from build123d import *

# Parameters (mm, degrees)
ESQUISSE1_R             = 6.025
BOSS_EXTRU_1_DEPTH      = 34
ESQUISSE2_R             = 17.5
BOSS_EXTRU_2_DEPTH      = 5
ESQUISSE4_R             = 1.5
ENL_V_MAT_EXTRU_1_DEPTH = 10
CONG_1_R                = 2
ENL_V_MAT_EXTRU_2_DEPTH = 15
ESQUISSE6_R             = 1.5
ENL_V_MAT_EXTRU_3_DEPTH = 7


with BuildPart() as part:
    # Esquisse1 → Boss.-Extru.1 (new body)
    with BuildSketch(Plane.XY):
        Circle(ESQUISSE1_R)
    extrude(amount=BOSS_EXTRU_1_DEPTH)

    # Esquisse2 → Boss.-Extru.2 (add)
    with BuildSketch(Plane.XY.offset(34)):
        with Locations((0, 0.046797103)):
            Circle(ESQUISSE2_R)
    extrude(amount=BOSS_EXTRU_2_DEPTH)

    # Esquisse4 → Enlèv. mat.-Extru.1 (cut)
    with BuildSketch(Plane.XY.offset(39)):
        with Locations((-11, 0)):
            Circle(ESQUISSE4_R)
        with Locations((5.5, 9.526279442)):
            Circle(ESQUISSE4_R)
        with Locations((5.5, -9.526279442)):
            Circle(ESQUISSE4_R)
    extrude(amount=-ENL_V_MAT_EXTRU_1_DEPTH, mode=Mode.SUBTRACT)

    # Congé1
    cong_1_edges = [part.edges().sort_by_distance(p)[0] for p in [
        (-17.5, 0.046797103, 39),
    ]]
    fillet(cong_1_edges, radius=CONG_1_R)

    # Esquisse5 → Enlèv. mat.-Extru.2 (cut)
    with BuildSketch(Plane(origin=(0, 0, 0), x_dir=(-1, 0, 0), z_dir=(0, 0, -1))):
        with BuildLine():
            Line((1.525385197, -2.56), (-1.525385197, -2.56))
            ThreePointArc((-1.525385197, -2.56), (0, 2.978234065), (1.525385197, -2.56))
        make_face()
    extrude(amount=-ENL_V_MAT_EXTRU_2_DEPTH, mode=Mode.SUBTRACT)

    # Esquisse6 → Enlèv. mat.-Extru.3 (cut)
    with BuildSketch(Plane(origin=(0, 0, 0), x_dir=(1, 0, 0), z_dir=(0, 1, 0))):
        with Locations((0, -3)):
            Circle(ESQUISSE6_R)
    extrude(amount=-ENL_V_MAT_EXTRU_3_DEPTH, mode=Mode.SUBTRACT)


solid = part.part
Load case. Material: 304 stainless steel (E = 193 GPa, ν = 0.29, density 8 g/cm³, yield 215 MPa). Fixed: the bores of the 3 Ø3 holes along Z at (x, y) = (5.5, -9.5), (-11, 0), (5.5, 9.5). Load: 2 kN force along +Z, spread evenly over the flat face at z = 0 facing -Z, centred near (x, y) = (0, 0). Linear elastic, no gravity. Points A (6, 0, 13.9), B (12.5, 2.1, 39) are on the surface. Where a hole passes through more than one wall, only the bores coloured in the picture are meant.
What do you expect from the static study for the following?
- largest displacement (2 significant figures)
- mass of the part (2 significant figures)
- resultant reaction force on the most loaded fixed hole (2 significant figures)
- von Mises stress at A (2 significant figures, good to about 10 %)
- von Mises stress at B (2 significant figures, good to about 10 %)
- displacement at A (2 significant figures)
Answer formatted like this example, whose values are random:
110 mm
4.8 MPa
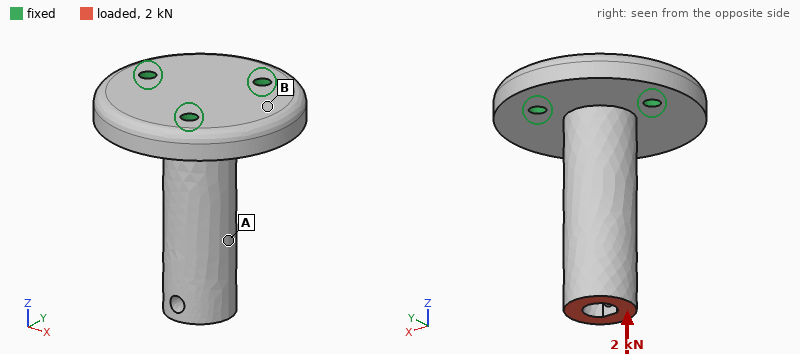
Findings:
6.5 µm
64 g
680 N
22 MPa
10 MPa
3.8 µm
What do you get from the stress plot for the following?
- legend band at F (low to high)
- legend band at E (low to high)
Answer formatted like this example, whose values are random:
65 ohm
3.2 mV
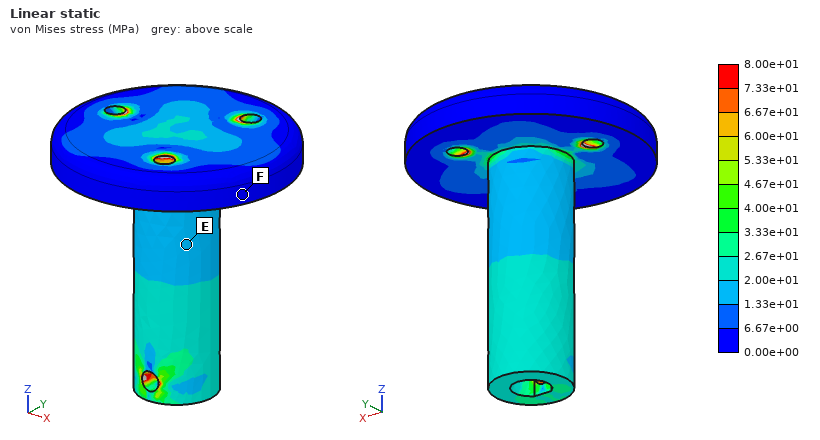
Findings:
0.00e+00 to 6.67e+00 MPa
1.33e+01 to 2.00e+01 MPa
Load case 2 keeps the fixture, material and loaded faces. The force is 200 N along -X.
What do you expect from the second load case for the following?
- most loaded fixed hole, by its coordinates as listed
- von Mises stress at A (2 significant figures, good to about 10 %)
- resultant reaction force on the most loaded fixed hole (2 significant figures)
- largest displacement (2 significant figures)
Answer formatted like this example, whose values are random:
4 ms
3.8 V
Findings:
(-11, 0)
18 MPa
440 N
22 µm
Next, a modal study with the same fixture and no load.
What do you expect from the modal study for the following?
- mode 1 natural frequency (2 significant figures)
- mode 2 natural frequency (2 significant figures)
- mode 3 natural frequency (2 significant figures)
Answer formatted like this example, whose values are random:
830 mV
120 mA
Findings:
5900 Hz
5900 Hz
22 kHz
